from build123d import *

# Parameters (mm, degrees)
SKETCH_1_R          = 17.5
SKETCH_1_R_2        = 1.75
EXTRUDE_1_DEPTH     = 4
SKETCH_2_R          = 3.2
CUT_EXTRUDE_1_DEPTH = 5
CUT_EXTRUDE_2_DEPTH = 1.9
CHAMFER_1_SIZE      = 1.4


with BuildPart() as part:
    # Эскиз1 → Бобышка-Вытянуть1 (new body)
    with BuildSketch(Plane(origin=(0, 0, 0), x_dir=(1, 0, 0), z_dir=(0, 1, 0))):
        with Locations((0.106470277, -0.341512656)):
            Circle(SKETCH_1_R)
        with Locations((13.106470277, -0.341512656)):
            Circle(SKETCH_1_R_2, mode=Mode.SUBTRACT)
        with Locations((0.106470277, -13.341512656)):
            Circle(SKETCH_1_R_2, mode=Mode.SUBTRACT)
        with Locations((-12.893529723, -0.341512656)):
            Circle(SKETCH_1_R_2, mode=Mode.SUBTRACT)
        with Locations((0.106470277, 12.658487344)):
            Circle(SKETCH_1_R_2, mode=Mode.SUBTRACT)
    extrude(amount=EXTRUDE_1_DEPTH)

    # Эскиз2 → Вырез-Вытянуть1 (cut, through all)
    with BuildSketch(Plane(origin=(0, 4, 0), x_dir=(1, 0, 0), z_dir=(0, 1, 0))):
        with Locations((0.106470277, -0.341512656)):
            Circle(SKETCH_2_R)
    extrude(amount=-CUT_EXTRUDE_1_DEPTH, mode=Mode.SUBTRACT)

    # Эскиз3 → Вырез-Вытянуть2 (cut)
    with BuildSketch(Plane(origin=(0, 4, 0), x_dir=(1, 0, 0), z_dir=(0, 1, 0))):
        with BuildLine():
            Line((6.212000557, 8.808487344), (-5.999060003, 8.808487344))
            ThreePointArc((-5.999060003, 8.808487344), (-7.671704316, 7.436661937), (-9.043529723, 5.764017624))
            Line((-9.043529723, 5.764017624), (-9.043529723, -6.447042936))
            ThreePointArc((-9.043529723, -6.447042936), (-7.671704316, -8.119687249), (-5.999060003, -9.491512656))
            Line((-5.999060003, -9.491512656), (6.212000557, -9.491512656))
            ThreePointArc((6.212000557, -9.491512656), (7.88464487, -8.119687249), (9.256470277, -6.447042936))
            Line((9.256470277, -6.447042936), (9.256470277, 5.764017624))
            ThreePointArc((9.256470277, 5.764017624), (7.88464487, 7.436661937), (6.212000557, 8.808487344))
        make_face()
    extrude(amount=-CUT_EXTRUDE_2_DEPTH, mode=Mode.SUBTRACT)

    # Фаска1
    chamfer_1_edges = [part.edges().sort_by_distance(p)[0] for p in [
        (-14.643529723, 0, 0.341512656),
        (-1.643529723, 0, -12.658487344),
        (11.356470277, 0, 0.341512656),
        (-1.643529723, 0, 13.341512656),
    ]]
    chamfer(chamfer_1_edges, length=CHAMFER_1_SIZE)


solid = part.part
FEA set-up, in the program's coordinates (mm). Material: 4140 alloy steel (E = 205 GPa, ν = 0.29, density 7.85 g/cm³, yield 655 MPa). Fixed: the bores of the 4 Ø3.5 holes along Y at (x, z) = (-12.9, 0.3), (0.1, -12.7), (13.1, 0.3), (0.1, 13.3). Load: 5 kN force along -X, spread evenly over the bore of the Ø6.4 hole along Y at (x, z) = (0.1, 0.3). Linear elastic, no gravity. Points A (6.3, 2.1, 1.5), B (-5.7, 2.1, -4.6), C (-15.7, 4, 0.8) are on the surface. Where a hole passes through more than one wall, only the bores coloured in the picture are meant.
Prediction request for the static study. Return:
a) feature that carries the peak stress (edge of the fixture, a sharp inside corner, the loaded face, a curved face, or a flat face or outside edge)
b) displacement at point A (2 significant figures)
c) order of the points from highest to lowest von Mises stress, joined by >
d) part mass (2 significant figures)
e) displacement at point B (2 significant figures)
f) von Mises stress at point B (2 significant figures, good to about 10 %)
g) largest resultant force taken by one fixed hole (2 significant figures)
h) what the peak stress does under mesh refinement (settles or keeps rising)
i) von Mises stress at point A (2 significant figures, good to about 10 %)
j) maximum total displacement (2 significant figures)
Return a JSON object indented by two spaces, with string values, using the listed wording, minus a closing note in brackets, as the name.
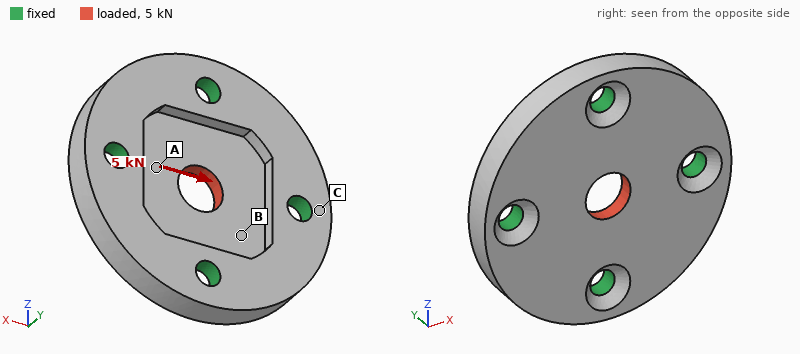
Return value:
{
  "feature that carries the peak stress": "edge of the fixture",
  "displacement at point A": "3.8 µm",
  "order of the points from highest to lowest von Mises stress, joined by >": "A > B > C",
  "part mass": "23 g",
  "displacement at point B": "2.9 µm",
  "von Mises stress at point B": "77 MPa",
  "largest resultant force taken by one fixed hole": "1.5 kN",
  "what the peak stress does under mesh refinement": "keeps rising",
  "von Mises stress at point A": "120 MPa",
  "maximum total displacement": "5.7 µm"
}
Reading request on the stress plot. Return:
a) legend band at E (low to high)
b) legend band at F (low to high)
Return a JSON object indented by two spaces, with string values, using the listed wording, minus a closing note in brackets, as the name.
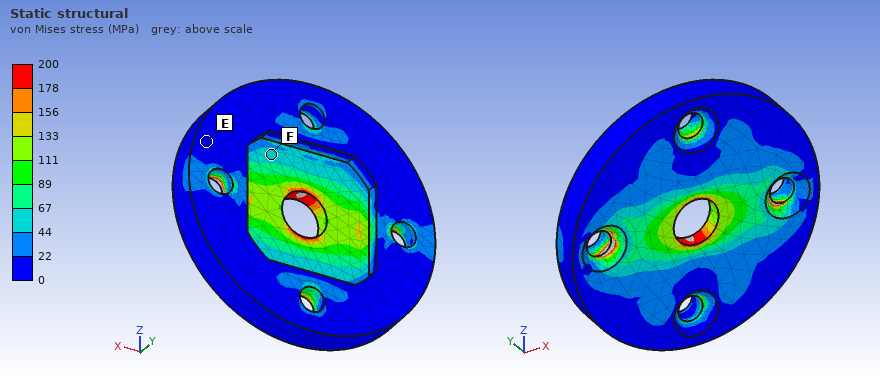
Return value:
{
  "legend band at E": "0 to 22 MPa",
  "legend band at F": "44 to 67 MPa"
}
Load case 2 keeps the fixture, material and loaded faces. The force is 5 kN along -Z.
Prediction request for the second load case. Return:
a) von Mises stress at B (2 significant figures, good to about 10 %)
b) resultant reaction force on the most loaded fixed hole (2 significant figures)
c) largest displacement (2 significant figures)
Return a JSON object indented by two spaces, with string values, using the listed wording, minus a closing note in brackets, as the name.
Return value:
{
  "von Mises stress at B": "67 MPa",
  "resultant reaction force on the most loaded fixed hole": "1.5 kN",
  "largest displacement": "5.7 µm"
}
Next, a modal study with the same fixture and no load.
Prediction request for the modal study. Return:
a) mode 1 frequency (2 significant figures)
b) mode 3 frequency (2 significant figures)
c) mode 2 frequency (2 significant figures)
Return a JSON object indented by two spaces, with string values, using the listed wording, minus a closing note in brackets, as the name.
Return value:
{
  "mode 1 frequency": "31 kHz",
  "mode 3 frequency": "33 kHz",
  "mode 2 frequency": "33 kHz"
}
